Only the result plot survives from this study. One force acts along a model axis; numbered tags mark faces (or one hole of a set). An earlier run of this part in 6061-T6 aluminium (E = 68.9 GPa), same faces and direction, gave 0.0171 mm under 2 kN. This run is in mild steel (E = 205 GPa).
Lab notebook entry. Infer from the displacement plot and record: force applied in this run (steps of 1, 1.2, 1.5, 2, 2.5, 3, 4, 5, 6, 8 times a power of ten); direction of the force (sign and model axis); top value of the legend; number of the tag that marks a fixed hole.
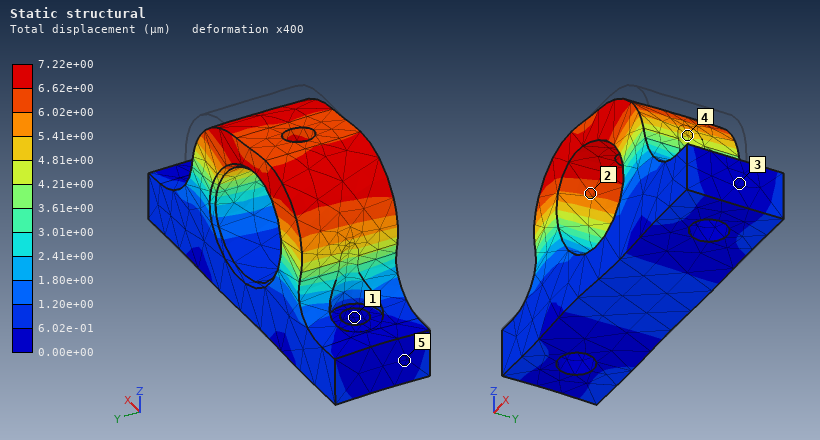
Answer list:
2.5 kN
-X
7.22e+00 µm
1
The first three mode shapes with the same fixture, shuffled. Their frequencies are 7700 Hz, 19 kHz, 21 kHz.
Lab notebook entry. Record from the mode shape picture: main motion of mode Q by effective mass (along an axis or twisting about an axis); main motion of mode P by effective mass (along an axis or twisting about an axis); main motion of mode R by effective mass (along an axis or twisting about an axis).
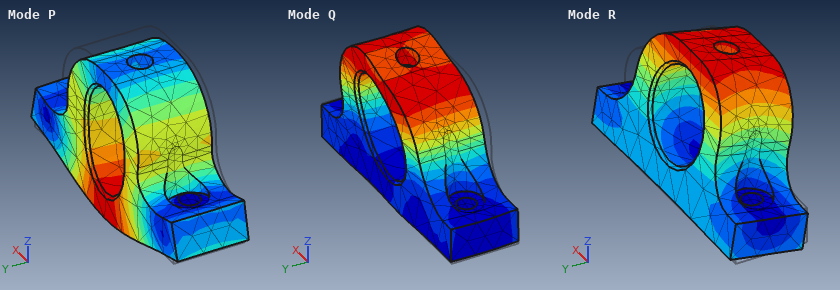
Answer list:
along X
along Z
along Y
